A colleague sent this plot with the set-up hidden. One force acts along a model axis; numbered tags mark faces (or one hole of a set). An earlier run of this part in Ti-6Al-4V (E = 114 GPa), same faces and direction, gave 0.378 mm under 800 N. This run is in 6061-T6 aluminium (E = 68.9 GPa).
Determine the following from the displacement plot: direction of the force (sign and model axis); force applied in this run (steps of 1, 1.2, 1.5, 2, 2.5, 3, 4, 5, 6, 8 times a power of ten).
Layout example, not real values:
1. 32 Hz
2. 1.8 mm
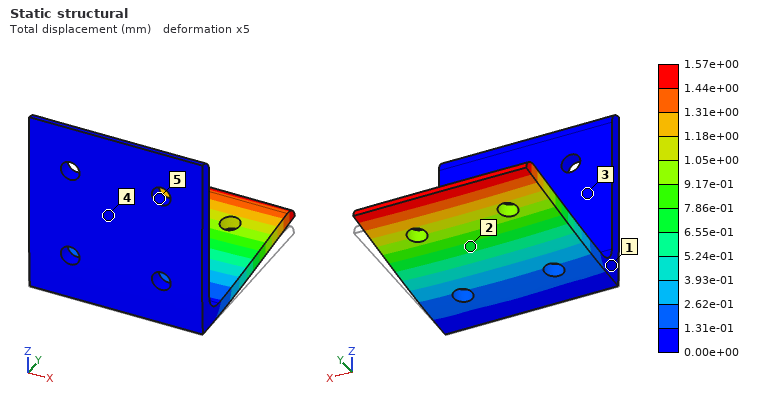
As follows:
1. +Z
2. 2 kN
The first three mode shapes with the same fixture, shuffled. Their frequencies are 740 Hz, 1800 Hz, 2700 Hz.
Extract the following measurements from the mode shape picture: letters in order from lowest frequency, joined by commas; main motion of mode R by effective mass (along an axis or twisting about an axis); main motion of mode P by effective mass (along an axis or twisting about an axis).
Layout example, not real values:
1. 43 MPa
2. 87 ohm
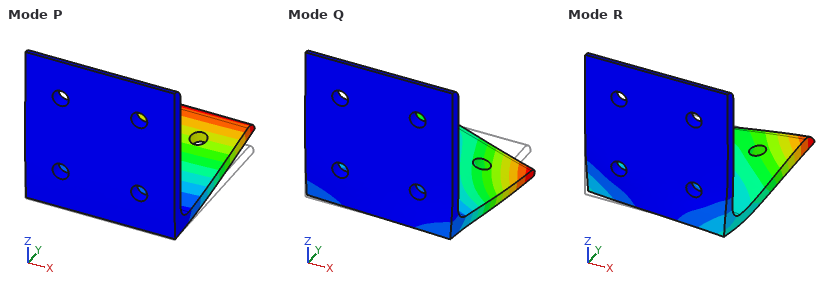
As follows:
1. P, Q, R
2. along X
3. along Z
